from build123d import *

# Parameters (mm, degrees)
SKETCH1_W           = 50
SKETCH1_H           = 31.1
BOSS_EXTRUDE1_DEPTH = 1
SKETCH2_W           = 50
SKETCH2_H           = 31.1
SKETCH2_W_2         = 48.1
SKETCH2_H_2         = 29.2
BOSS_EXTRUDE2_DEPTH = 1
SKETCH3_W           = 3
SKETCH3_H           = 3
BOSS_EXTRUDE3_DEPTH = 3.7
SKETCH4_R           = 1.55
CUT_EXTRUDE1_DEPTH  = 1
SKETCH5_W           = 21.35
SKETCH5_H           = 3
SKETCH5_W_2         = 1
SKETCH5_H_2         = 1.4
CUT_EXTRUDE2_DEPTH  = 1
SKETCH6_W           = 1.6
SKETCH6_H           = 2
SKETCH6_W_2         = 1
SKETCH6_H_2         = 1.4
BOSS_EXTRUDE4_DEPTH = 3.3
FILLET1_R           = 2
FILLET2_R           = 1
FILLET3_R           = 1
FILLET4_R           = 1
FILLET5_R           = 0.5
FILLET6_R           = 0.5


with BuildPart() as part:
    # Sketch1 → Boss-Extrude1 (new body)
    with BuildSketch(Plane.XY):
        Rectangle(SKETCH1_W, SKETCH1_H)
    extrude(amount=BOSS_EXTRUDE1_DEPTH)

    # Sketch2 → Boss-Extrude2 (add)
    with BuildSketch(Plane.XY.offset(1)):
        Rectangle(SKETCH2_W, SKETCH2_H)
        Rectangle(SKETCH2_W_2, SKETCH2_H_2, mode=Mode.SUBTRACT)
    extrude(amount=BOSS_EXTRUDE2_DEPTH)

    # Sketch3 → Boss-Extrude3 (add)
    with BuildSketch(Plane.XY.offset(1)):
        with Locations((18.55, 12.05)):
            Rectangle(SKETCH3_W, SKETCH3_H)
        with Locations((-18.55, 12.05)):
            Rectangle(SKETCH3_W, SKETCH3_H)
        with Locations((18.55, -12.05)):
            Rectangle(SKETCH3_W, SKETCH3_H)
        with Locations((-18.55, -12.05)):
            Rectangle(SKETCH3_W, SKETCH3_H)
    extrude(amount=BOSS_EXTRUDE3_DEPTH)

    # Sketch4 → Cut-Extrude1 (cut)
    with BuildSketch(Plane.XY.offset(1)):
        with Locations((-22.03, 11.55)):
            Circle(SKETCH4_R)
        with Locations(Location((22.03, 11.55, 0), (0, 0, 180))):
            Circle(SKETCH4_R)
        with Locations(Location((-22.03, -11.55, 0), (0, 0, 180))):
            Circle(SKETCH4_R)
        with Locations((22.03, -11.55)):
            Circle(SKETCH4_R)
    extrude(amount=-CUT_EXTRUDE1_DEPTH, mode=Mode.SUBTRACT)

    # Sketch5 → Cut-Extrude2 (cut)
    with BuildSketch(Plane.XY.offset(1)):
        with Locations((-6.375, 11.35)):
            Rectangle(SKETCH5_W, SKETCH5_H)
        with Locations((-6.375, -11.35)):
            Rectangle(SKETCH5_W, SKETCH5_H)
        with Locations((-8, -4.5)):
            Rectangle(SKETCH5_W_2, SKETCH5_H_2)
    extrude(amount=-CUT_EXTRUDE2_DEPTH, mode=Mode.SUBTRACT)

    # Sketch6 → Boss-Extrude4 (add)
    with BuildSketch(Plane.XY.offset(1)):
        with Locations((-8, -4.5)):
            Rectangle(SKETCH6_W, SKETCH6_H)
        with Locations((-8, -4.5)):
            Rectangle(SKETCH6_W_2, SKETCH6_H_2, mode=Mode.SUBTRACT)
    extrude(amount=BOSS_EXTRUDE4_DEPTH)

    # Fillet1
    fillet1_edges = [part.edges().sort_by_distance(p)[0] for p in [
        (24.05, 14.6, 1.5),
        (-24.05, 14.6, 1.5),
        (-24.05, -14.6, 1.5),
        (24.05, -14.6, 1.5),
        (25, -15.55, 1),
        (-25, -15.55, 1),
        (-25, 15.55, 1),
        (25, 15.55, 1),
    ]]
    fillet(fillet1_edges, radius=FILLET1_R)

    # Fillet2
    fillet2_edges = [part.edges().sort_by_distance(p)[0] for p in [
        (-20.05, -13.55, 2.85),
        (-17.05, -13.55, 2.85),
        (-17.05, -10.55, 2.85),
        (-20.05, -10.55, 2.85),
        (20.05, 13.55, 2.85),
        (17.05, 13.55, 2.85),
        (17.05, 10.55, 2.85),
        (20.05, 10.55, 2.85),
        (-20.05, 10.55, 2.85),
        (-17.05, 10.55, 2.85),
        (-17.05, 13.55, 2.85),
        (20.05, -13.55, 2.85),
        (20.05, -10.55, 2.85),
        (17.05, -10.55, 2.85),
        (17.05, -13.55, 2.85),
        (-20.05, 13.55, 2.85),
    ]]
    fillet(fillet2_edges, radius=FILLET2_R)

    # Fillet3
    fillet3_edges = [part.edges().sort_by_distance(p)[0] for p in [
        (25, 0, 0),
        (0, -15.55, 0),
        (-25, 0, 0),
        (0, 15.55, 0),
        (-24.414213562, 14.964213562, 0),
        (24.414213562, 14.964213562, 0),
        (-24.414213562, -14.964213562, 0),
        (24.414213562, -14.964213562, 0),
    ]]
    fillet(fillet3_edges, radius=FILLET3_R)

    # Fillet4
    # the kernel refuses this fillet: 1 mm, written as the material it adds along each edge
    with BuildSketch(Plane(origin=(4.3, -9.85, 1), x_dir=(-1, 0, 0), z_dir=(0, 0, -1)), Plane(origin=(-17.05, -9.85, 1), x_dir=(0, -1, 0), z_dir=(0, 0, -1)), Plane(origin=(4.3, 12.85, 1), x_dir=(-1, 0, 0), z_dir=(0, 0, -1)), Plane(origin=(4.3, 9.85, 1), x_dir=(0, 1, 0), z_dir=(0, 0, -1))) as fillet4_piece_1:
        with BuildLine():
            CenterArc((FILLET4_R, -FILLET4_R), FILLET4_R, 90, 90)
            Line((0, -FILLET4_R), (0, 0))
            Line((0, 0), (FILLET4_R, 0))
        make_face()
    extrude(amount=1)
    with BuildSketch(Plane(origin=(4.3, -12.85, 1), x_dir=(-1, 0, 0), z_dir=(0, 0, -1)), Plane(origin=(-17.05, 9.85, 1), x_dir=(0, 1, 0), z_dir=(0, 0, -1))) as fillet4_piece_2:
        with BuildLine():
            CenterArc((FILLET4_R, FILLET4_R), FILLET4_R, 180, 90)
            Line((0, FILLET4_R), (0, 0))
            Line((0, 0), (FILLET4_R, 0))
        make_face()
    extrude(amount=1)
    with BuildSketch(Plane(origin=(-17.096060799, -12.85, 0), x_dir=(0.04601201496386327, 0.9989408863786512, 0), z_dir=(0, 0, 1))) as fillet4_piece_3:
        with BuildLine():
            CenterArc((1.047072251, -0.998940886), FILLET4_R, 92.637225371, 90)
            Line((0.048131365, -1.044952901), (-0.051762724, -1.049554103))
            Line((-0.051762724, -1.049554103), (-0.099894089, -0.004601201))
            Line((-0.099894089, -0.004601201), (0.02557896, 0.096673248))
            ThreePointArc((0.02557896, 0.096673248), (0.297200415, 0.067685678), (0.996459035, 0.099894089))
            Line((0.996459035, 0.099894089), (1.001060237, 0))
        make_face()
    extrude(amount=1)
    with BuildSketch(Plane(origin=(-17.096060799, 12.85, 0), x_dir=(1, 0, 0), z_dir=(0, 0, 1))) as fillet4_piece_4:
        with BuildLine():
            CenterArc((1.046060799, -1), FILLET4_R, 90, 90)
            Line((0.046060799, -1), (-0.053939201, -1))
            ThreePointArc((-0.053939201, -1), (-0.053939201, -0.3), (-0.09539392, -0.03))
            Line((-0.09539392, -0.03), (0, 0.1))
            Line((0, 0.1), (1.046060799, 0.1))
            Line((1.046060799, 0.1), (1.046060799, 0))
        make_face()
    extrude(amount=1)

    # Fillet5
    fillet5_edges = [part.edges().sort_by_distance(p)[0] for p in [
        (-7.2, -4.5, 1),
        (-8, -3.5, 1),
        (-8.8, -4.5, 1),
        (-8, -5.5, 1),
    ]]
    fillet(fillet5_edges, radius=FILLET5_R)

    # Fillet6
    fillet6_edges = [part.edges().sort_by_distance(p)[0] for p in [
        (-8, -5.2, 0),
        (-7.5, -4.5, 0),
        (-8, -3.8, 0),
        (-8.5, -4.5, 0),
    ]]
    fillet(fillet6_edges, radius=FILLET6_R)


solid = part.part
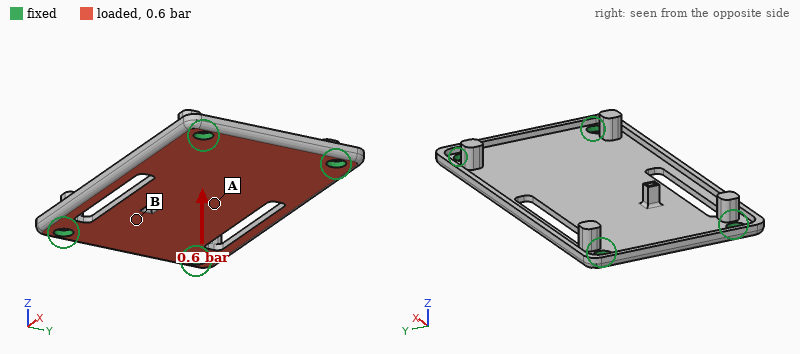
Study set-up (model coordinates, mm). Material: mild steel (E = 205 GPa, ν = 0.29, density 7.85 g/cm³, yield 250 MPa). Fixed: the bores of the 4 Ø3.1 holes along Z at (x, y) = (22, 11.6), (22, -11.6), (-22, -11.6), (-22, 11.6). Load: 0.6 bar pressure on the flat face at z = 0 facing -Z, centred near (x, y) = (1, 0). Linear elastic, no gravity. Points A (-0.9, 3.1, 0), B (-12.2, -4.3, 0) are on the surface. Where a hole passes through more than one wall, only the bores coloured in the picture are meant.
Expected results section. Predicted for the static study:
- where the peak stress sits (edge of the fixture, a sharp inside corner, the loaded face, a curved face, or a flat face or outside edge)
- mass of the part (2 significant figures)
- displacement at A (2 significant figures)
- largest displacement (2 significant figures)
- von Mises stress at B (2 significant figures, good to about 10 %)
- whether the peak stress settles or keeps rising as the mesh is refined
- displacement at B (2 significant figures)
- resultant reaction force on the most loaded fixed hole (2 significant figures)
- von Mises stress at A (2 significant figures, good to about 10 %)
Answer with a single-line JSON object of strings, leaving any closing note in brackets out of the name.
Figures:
{"where the peak stress sits": "edge of the fixture", "mass of the part": "13 g", "displacement at A": "25 µm", "largest displacement": "25 µm", "von Mises stress at B": "8.5 MPa", "whether the peak stress settles or keeps rising as the mesh is refined": "keeps rising", "displacement at B": "14 µm", "resultant reaction force on the most loaded fixed hole": "20 N", "von Mises stress at A": "19 MPa"}
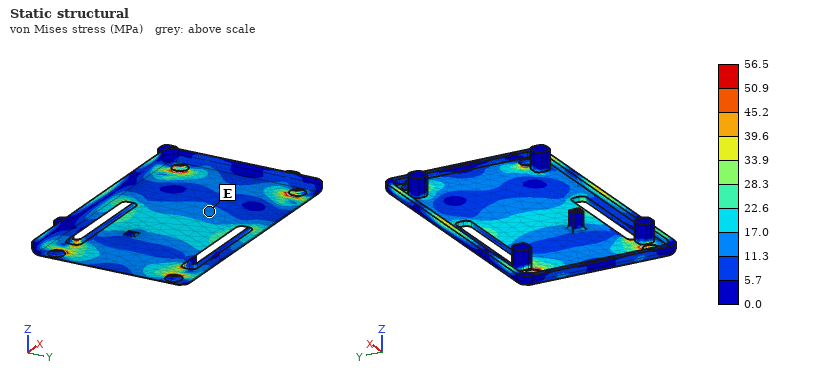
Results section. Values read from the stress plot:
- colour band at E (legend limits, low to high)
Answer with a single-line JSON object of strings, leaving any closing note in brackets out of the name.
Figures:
{"colour band at E": "11.3 to 17.0 MPa"}
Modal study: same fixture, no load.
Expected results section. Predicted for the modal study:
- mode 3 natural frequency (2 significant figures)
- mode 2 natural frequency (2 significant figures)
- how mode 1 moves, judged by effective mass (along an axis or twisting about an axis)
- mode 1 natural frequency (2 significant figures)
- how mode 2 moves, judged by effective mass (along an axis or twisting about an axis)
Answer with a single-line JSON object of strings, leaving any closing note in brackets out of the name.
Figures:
{"mode 3 natural frequency": "6700 Hz", "mode 2 natural frequency": "5000 Hz", "how mode 1 moves, judged by effective mass": "along Z", "mode 1 natural frequency": "3200 Hz", "how mode 2 moves, judged by effective mass": "twisting about X"}
